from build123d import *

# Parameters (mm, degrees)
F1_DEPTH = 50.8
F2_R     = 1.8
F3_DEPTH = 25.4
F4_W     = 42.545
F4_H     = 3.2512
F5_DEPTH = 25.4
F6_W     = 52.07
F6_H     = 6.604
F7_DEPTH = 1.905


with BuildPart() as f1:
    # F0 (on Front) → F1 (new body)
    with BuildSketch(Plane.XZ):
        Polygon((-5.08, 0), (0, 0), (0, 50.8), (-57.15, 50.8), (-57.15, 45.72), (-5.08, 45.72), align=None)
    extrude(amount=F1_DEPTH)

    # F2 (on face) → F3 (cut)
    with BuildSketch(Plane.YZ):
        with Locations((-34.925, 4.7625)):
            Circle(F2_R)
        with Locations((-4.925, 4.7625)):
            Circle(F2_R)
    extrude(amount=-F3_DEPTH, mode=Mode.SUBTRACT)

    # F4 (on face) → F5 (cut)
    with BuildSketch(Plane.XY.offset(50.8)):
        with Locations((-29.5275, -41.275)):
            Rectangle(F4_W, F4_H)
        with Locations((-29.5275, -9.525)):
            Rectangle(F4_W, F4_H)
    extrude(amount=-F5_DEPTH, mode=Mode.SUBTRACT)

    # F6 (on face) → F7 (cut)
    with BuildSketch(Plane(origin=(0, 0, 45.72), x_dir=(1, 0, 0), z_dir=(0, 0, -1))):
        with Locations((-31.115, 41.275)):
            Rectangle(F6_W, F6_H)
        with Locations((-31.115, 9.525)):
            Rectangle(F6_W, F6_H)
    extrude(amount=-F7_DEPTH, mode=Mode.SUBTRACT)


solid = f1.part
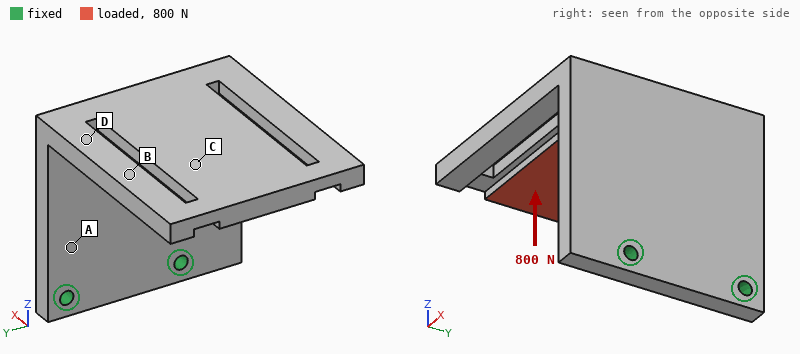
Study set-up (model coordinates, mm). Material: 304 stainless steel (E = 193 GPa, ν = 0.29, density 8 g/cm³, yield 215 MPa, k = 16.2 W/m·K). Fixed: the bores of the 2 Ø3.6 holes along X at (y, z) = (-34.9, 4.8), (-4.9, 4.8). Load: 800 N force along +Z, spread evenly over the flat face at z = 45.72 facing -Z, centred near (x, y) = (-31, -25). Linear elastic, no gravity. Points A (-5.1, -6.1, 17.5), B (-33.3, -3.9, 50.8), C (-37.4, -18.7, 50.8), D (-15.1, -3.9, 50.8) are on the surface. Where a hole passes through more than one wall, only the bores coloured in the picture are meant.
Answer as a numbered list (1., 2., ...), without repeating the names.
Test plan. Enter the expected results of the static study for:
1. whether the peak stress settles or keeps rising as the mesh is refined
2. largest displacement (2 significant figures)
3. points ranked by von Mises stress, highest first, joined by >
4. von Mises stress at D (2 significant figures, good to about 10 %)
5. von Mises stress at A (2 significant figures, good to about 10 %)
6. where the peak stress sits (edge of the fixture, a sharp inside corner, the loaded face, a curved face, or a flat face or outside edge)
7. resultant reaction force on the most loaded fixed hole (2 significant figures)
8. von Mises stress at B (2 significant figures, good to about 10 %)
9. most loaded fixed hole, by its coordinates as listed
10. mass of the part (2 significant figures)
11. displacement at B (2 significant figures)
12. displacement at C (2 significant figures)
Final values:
1. keeps rising
2. 0.75 mm
3. A > D > B > C
4. 73 MPa
5. 110 MPa
6. edge of the fixture
7. 540 N
8. 38 MPa
9. (-34.9, 4.8)
10. 190 g
11. 0.44 mm
12. 0.50 mm
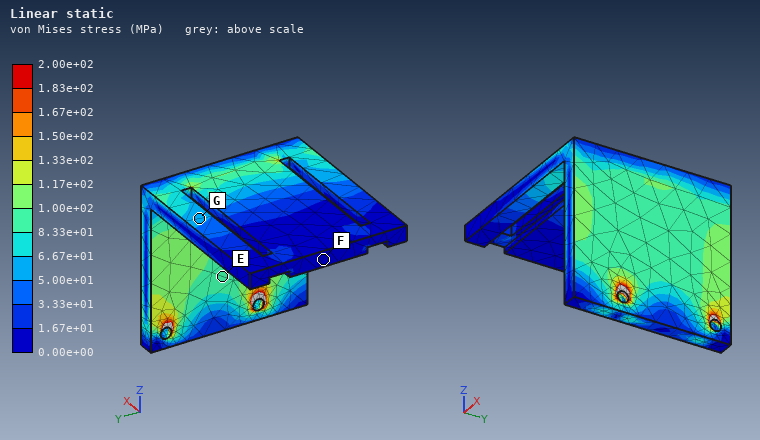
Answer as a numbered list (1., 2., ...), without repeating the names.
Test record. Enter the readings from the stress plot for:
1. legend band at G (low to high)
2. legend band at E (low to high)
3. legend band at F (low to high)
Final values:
1. 5.00e+01 to 6.67e+01 MPa
2. 8.33e+01 to 1.00e+02 MPa
3. 0.00e+00 to 1.67e+01 MPa
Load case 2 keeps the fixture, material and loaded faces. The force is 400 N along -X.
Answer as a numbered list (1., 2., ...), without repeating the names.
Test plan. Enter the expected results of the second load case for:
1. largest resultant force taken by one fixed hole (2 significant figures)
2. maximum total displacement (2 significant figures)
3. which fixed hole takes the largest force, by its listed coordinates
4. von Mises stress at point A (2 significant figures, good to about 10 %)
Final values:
1. 280 N
2. 0.22 mm
3. (-34.9, 4.8)
4. 54 MPa
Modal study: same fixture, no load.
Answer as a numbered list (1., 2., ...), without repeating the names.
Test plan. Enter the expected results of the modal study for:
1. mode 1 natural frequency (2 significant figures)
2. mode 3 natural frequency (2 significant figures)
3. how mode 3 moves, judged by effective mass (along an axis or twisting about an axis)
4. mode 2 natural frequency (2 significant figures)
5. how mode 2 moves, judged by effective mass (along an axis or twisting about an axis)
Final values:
1. 570 Hz
2. 1500 Hz
3. along X
4. 1000 Hz
5. along Y
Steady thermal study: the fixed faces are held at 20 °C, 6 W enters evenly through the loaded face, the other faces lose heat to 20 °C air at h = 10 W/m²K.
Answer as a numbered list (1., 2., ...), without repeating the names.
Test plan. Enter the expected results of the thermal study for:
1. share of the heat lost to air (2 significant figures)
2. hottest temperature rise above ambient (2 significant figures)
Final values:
1. 56 %
2. 67 K
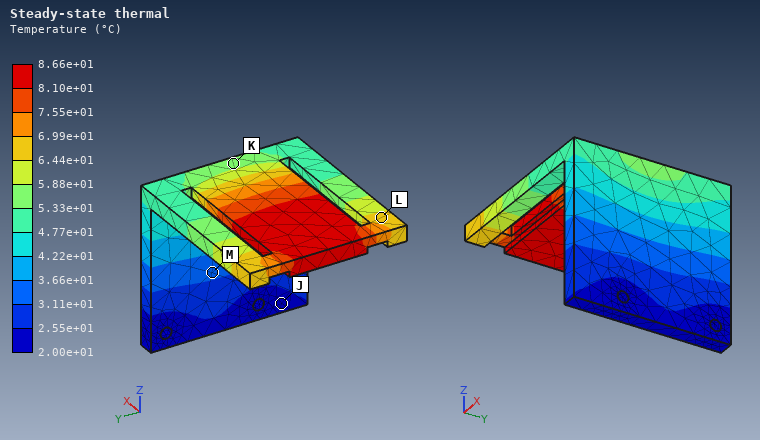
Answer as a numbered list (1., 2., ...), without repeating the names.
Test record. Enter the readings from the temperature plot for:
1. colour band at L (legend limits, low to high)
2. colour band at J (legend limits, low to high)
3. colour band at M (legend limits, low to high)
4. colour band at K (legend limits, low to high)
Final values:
1. 6.44e+01 to 6.99e+01 °C
2. 2.00e+01 to 2.55e+01 °C
3. 3.11e+01 to 3.66e+01 °C
4. 5.33e+01 to 5.88e+01 °C
